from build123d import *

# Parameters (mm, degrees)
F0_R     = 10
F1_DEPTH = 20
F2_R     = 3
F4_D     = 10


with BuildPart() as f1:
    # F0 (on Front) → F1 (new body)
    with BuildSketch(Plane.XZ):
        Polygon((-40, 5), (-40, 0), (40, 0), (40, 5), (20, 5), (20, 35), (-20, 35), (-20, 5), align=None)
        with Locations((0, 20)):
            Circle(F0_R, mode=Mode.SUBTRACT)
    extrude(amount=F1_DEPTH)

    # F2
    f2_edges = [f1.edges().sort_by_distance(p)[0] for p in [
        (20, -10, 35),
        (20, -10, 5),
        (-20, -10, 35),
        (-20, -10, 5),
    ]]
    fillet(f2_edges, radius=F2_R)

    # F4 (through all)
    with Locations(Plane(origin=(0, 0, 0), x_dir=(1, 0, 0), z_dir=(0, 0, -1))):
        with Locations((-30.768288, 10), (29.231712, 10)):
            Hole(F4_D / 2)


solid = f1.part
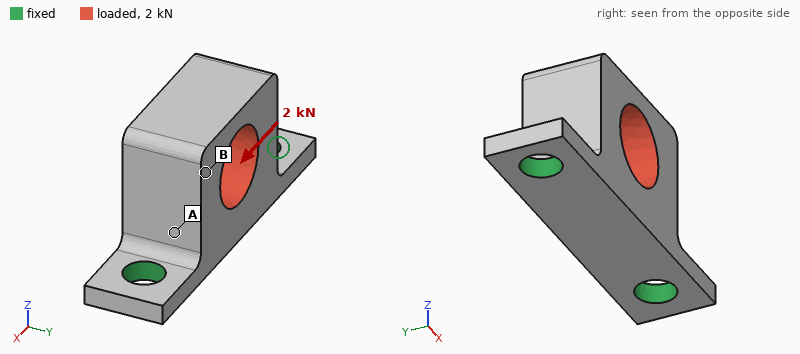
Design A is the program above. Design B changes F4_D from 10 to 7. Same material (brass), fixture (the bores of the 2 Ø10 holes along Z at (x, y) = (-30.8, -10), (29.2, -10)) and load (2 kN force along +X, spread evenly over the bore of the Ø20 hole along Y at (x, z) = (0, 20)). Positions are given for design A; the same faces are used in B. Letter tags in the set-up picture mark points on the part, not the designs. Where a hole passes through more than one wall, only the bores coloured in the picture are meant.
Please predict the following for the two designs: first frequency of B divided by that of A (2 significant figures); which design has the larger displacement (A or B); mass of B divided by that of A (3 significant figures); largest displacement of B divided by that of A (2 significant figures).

0.84
B
1.02
1.2
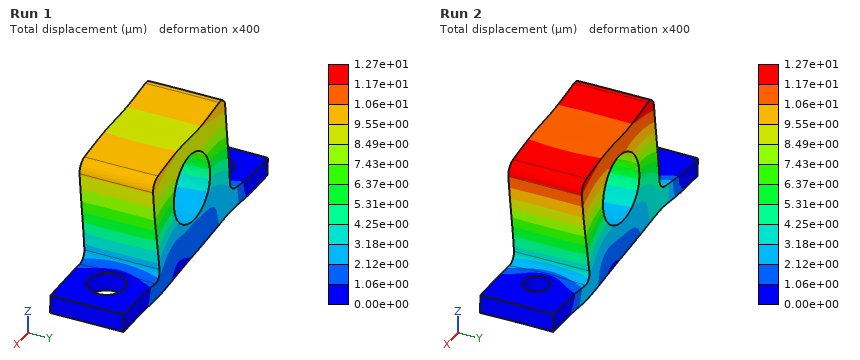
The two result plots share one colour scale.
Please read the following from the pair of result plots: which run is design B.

Run 2
